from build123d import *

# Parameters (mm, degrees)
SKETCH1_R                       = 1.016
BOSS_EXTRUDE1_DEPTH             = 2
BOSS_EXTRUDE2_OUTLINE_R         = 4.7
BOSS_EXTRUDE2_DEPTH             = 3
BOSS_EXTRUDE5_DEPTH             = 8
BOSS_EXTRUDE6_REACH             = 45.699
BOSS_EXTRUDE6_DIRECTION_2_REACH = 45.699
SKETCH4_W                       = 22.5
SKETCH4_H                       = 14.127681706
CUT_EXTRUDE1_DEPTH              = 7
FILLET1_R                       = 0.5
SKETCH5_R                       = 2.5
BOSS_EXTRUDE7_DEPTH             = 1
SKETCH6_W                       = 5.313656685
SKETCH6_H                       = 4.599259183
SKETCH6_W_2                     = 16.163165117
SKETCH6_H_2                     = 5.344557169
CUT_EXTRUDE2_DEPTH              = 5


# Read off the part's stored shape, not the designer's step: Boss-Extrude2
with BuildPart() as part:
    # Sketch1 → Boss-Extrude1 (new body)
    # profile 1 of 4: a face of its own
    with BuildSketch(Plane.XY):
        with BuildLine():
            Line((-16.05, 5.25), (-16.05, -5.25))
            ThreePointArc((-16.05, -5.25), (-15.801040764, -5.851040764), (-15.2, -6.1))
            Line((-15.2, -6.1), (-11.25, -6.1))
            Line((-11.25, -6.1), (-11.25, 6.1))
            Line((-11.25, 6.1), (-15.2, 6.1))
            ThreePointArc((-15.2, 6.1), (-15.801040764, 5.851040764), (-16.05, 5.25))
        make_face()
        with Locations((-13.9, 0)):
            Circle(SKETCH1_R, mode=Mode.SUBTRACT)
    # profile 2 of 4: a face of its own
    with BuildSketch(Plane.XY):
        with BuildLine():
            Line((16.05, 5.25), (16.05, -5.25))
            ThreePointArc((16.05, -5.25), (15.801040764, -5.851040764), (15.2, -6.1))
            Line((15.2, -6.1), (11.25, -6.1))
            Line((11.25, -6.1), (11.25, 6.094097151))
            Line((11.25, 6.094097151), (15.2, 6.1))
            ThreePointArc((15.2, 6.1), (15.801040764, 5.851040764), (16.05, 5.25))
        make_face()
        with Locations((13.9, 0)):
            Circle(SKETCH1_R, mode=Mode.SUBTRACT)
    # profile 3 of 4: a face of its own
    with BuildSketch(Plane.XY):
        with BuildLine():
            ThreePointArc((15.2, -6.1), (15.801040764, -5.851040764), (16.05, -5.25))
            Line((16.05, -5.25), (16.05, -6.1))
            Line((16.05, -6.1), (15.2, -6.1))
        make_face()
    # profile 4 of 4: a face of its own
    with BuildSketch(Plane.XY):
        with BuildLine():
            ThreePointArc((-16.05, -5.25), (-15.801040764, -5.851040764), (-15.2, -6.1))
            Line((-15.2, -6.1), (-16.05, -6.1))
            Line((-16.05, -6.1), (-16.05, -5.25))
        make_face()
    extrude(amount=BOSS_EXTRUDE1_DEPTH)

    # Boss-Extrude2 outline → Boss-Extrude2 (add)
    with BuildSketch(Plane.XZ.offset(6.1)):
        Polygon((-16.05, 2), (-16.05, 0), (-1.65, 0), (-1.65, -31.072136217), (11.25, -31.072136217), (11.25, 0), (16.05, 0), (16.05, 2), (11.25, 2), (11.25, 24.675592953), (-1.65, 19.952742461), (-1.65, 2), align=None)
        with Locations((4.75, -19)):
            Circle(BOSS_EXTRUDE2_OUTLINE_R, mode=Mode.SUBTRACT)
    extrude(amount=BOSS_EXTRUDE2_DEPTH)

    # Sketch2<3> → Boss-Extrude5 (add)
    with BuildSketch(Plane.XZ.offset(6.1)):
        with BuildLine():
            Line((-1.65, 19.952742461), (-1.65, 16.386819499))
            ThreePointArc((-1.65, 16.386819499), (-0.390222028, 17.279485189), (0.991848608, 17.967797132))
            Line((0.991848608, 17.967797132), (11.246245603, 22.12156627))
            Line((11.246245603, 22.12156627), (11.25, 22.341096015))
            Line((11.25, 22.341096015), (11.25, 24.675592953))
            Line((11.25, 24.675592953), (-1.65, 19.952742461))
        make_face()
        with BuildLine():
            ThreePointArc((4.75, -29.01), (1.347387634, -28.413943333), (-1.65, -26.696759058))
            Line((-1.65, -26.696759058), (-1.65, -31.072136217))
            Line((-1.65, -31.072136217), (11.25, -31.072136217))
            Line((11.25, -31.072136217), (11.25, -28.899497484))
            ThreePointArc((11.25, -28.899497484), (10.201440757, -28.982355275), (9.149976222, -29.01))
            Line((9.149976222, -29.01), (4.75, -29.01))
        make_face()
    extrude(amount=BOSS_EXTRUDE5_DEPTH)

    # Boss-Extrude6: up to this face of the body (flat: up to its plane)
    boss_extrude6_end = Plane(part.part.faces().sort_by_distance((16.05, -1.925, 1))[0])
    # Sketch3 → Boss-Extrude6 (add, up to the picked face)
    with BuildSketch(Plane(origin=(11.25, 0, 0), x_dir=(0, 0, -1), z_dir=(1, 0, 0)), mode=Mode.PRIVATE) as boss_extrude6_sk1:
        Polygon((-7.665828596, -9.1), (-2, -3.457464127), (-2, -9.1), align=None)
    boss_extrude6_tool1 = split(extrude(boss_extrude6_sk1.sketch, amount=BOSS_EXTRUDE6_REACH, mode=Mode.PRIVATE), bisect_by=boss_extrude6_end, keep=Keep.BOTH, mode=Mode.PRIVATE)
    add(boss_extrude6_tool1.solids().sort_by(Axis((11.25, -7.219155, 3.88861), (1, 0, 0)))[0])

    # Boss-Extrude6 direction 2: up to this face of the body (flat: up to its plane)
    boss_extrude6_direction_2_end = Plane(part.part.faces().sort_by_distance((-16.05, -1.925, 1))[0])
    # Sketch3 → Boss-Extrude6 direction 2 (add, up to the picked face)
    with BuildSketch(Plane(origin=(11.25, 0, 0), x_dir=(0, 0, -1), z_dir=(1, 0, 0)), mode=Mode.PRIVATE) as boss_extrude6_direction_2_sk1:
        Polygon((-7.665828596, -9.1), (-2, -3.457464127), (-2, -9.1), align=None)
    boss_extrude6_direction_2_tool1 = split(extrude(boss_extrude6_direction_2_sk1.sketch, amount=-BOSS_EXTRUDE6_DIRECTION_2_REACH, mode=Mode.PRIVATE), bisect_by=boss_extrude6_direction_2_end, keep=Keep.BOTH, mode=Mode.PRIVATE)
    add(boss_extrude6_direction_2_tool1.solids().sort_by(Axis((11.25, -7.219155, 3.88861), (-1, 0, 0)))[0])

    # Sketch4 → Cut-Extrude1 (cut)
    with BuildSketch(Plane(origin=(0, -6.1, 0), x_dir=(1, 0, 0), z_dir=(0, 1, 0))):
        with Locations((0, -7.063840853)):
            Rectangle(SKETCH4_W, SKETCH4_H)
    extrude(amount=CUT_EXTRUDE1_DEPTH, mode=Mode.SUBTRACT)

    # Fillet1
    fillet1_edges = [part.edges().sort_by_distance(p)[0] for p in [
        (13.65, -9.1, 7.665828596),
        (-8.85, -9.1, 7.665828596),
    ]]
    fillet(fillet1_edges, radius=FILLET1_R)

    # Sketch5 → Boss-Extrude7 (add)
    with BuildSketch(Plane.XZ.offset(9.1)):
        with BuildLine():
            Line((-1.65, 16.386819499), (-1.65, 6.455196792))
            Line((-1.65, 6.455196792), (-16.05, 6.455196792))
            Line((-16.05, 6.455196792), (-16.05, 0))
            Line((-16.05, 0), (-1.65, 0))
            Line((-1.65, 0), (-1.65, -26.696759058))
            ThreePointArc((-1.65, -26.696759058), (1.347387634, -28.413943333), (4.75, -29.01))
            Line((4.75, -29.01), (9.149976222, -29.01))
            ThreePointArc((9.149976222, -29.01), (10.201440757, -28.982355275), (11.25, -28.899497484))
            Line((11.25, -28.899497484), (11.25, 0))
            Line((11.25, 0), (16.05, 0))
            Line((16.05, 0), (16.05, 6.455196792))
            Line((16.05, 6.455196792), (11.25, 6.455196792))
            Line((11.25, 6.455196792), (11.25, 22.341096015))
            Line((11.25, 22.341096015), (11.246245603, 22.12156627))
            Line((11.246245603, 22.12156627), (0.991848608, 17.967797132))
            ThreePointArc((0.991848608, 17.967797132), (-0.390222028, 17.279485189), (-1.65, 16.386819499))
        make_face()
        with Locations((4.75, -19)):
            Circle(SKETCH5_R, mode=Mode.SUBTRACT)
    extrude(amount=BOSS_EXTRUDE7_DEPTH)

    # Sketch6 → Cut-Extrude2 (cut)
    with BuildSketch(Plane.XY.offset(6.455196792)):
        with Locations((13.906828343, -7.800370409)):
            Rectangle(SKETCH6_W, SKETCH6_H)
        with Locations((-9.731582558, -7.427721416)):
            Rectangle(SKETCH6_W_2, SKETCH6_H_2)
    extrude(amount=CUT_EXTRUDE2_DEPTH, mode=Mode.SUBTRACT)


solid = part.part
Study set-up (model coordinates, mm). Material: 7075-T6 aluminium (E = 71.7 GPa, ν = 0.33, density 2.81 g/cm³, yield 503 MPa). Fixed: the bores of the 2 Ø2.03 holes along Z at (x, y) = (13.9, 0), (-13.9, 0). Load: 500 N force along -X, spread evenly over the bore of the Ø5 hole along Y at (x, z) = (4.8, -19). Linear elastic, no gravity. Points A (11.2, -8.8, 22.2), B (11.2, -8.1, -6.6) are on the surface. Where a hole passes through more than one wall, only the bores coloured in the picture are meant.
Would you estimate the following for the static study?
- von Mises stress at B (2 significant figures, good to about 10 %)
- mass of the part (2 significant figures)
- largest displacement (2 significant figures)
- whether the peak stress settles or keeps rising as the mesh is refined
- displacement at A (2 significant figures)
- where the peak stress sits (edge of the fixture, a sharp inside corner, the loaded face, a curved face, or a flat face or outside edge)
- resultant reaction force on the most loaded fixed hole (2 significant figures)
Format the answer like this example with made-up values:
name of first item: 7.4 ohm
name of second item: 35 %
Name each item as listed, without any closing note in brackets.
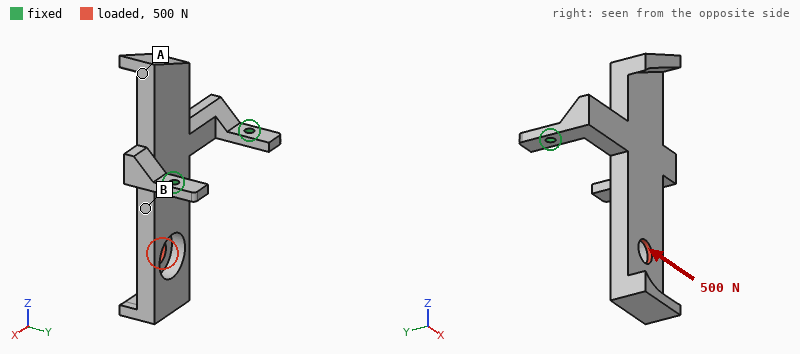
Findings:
von Mises stress at B: 58 MPa
mass of the part: 9.9 g
largest displacement: 0.37 mm
whether the peak stress settles or keeps rising as the mesh is refined: keeps rising
displacement at A: 0.15 mm
where the peak stress sits: edge of the fixture
resultant reaction force on the most loaded fixed hole: 470 N
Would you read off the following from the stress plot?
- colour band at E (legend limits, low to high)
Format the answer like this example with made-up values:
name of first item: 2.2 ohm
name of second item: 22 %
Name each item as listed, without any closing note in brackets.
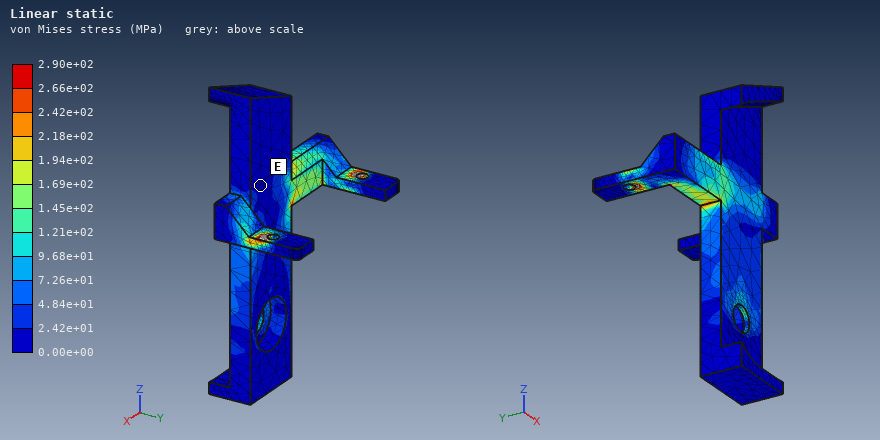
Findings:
colour band at E: 0.00e+00 to 2.42e+01 MPa
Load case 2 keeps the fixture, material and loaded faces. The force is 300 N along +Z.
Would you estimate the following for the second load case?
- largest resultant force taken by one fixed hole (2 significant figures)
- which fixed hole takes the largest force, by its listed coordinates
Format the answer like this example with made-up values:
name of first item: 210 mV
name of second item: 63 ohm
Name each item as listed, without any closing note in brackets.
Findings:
largest resultant force taken by one fixed hole: 200 N
which fixed hole takes the largest force, by its listed coordinates: (13.9, 0)
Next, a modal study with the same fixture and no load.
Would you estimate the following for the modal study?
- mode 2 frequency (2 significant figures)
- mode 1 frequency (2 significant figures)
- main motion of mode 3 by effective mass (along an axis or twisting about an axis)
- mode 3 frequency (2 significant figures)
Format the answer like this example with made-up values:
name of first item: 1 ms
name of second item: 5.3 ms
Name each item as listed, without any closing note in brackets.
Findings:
mode 2 frequency: 3400 Hz
mode 1 frequency: 910 Hz
main motion of mode 3 by effective mass: along Y
mode 3 frequency: 3800 Hz
